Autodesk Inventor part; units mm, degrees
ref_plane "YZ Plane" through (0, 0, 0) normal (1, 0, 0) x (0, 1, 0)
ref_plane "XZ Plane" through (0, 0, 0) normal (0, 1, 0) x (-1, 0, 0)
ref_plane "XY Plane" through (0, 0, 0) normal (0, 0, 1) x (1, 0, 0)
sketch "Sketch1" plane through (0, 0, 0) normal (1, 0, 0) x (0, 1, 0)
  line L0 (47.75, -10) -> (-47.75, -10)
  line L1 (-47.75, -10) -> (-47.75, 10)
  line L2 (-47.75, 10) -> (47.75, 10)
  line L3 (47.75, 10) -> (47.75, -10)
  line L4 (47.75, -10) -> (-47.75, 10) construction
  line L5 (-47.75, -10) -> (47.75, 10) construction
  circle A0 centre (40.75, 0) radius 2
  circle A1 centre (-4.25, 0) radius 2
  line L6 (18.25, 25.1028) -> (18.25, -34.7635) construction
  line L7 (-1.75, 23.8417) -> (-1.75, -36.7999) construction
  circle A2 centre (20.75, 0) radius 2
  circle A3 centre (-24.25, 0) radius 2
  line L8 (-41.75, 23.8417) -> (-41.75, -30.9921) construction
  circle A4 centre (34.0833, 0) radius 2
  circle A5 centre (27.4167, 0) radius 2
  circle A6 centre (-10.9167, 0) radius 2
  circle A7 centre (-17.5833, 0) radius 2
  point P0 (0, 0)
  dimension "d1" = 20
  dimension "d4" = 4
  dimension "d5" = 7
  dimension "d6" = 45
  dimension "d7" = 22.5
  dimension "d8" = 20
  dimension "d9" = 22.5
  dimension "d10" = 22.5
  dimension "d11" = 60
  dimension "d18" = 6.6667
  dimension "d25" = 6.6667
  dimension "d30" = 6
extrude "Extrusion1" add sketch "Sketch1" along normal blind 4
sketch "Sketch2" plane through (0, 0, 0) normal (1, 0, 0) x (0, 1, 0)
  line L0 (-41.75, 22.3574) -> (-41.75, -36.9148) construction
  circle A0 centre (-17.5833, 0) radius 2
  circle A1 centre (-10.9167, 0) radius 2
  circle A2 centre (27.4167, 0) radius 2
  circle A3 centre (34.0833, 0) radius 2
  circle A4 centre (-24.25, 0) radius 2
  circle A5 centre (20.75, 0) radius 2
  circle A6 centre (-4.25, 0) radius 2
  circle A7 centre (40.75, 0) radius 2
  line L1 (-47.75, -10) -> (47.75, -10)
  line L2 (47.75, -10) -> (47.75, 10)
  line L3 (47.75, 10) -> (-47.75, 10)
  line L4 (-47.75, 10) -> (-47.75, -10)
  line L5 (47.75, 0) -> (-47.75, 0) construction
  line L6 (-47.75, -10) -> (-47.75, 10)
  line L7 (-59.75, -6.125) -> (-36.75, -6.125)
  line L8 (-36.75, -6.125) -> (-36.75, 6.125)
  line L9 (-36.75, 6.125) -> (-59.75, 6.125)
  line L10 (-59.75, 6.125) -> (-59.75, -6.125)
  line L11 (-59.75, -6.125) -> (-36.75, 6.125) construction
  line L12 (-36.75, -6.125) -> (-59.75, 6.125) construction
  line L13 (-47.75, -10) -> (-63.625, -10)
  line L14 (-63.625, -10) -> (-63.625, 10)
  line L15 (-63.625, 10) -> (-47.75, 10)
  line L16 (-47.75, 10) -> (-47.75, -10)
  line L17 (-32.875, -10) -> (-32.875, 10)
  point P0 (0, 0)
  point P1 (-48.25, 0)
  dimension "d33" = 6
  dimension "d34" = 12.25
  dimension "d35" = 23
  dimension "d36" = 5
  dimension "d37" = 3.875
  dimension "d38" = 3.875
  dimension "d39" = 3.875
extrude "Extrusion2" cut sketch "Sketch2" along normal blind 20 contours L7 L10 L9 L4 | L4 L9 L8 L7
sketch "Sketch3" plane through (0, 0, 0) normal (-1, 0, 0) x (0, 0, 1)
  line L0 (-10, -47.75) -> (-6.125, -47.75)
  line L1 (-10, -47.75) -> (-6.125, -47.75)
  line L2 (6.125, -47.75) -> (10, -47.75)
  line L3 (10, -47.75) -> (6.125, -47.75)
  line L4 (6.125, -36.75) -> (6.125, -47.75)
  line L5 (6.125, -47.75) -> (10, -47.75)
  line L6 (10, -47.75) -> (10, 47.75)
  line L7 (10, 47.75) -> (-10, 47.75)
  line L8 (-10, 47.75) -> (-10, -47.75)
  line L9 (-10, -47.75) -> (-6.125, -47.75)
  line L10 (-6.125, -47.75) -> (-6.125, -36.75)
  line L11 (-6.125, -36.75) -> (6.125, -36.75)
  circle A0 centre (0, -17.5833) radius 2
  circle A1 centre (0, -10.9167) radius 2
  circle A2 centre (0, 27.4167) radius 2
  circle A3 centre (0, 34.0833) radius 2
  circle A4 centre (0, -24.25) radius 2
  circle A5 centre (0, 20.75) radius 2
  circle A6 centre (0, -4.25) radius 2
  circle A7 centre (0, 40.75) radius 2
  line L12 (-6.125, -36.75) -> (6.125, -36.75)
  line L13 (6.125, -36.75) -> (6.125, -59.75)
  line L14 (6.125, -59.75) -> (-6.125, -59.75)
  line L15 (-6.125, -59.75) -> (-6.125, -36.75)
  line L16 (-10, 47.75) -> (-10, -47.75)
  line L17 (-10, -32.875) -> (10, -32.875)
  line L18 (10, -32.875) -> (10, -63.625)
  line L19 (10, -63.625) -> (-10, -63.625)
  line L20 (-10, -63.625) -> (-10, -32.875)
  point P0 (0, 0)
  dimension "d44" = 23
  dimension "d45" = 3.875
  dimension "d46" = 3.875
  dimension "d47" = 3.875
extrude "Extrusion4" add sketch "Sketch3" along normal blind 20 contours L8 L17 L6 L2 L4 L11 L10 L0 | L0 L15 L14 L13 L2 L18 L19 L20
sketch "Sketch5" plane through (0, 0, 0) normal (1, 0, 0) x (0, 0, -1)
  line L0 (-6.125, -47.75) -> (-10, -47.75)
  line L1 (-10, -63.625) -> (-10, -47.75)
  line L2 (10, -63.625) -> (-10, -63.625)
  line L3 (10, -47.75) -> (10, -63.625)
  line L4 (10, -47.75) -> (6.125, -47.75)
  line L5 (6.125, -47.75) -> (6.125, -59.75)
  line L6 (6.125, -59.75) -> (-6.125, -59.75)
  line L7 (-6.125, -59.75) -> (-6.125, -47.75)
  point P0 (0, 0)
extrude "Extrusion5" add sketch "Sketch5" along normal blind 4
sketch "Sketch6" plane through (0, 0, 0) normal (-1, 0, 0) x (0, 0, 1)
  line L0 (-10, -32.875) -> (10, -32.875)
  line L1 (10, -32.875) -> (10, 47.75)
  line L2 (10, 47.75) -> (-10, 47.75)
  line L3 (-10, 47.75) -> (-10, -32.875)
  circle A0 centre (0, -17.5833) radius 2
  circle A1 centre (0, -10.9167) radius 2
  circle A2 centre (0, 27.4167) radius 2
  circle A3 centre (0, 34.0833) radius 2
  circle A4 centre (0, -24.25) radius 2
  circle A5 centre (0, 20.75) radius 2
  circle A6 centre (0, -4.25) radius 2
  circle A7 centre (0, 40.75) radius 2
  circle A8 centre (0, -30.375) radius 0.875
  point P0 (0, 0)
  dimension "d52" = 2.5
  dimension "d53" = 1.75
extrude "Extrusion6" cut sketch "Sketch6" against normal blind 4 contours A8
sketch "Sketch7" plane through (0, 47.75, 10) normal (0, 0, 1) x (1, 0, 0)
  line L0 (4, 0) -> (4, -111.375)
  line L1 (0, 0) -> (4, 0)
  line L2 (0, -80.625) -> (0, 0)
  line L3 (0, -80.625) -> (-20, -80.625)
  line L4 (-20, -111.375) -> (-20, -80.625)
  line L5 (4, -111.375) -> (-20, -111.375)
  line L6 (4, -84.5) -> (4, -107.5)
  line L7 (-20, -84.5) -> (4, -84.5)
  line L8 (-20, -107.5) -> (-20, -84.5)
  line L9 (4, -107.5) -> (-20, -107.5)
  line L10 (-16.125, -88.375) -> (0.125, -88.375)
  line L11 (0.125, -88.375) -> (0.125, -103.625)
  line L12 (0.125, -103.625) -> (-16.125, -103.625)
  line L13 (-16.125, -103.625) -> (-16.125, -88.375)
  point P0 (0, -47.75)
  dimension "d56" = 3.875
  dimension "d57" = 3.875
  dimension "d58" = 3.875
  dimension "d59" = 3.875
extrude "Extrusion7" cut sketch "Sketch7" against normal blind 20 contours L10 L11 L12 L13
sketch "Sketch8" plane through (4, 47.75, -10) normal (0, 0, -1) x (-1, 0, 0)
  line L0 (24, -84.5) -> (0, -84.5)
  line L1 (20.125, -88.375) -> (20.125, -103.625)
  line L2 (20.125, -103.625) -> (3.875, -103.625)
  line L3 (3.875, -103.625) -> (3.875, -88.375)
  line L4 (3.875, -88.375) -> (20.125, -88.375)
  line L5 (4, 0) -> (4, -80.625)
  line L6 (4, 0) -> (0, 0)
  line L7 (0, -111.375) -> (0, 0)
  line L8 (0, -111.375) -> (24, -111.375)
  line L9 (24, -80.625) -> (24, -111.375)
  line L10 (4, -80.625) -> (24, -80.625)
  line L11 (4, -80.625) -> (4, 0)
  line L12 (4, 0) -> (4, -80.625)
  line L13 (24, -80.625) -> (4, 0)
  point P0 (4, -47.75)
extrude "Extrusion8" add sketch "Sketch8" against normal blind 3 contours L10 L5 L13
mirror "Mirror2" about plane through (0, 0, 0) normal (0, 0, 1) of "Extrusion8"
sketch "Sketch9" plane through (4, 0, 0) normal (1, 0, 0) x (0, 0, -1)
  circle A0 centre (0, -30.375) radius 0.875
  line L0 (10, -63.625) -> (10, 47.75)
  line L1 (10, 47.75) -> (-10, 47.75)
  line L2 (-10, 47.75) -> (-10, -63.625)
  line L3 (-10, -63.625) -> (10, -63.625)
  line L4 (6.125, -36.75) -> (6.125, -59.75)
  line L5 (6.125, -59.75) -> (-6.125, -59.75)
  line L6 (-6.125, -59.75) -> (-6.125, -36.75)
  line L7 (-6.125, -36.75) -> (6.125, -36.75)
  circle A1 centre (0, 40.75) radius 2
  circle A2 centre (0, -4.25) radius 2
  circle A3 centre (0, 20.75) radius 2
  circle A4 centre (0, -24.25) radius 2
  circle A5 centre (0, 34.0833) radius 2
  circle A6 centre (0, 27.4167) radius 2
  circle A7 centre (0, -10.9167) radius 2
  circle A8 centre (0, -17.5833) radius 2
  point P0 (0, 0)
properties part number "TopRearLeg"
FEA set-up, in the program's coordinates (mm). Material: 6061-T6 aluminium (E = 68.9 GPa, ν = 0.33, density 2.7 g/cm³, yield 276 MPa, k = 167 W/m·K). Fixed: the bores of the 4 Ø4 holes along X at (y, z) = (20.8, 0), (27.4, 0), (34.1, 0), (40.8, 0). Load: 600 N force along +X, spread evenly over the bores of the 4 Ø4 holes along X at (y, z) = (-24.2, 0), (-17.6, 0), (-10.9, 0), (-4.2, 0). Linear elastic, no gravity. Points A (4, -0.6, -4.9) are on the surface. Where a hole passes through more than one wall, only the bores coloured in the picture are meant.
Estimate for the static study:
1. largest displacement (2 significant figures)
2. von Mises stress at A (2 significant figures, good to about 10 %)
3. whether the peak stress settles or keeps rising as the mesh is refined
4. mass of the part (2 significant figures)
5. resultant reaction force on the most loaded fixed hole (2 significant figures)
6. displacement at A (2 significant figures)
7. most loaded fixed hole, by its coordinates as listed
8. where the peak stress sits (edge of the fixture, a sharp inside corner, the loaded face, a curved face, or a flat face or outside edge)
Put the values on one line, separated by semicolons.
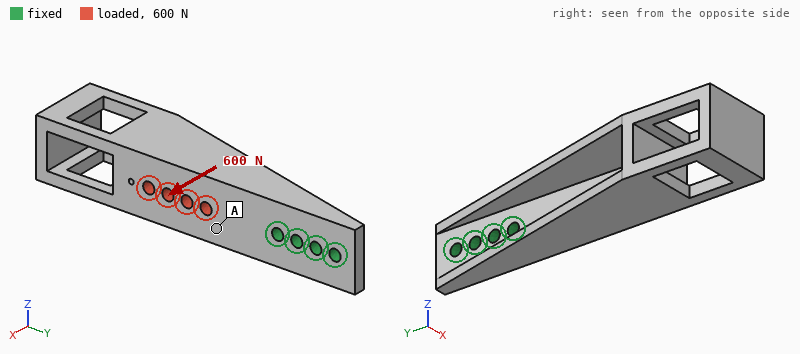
0.48 mm; 17 MPa; keeps rising; 46 g; 1.8 kN; 0.11 mm; (20.8, 0); edge of the fixture
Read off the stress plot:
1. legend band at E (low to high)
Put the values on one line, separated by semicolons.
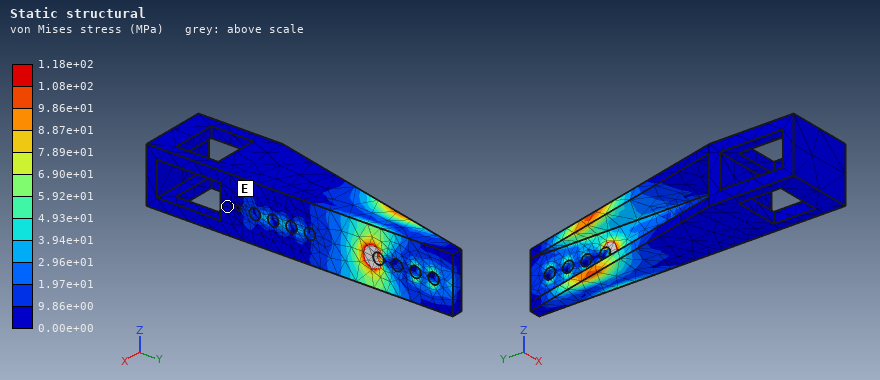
0.00e+00 to 9.86e+00 MPa
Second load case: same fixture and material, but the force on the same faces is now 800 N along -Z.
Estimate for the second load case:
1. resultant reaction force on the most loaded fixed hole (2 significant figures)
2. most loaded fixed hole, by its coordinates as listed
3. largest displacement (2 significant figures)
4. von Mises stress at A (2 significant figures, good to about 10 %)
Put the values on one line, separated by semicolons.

2.1 kN; (20.8, 0); 0.21 mm; 15 MPa
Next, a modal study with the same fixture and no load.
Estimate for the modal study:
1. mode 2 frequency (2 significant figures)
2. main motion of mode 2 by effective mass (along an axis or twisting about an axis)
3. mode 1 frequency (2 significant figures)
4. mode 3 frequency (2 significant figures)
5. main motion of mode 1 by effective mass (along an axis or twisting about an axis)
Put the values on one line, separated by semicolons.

1300 Hz; along Z; 900 Hz; 2300 Hz; along X
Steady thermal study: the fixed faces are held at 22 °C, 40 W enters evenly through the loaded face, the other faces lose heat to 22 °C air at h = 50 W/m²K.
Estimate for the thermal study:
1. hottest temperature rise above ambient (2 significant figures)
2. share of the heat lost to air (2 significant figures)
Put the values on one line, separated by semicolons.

47 K; 37 %
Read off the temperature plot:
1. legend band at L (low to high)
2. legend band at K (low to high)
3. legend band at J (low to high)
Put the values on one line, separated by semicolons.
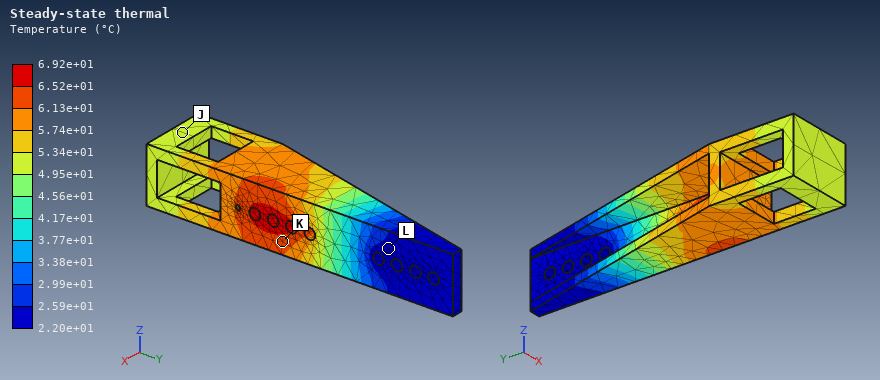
2.20e+01 to 2.59e+01 °C; 6.13e+01 to 6.52e+01 °C; 4.95e+01 to 5.34e+01 °C
